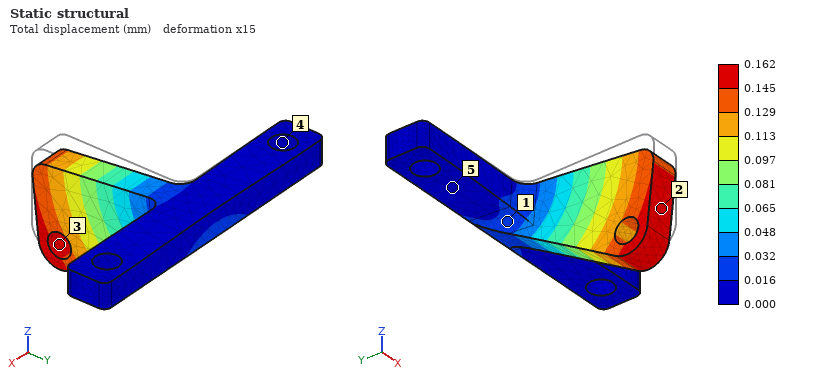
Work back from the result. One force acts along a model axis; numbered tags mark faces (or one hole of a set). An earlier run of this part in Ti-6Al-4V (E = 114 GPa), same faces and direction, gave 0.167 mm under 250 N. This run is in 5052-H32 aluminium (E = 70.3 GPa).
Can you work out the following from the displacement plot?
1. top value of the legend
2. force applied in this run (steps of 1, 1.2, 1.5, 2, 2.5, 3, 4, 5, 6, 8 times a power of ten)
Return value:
0.162 mm
150 N
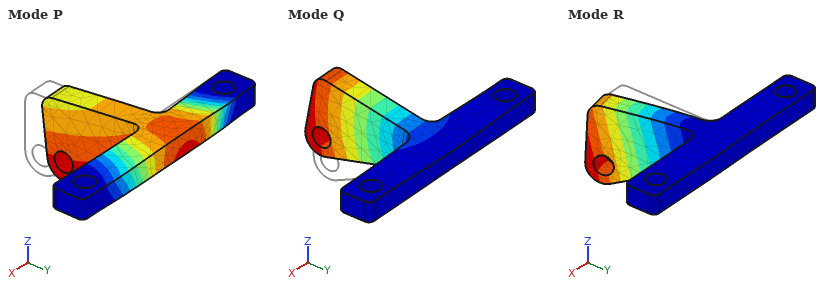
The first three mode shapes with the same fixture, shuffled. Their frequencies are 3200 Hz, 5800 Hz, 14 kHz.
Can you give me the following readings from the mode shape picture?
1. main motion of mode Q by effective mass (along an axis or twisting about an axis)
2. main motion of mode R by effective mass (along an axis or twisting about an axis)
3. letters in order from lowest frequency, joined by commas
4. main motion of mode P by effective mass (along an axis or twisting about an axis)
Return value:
along Z
along X
Q, R, P
along Y
